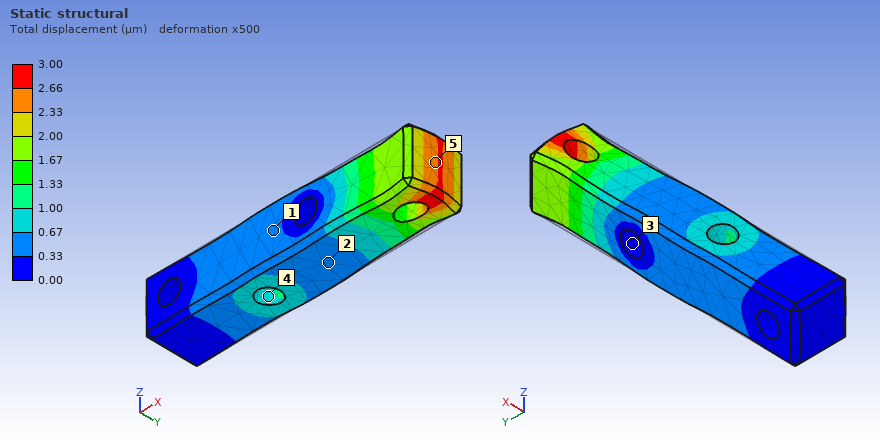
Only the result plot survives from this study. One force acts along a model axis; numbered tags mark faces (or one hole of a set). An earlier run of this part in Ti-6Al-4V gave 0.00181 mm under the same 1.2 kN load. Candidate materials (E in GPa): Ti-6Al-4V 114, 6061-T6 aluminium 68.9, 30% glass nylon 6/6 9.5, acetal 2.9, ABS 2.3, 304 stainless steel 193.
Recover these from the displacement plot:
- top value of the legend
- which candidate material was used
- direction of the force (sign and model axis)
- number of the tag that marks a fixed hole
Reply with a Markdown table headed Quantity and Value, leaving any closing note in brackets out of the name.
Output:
| Quantity | Value |
|---|---|
| top value of the legend | 3.00 µm |
| which candidate material was used | 6061-T6 aluminium |
| direction of the force | +X |
| number of the tag that marks a fixed hole | 3 |
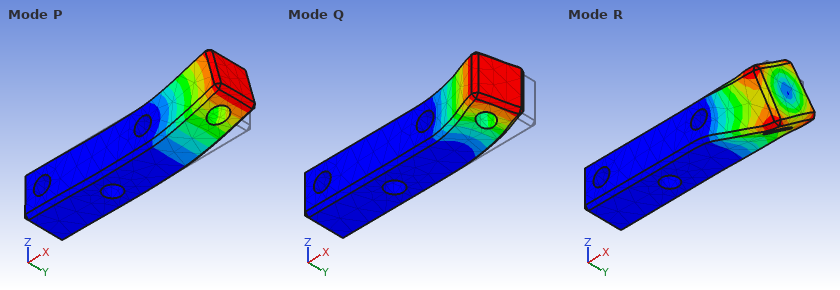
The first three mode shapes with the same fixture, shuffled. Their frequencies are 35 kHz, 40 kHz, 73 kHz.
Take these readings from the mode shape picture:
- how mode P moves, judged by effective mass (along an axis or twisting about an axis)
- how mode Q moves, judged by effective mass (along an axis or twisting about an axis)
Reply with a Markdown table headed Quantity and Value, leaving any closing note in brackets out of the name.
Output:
| Quantity | Value |
|---|---|
| how mode P moves, judged by effective mass | along Z |
| how mode Q moves, judged by effective mass | along Y |
